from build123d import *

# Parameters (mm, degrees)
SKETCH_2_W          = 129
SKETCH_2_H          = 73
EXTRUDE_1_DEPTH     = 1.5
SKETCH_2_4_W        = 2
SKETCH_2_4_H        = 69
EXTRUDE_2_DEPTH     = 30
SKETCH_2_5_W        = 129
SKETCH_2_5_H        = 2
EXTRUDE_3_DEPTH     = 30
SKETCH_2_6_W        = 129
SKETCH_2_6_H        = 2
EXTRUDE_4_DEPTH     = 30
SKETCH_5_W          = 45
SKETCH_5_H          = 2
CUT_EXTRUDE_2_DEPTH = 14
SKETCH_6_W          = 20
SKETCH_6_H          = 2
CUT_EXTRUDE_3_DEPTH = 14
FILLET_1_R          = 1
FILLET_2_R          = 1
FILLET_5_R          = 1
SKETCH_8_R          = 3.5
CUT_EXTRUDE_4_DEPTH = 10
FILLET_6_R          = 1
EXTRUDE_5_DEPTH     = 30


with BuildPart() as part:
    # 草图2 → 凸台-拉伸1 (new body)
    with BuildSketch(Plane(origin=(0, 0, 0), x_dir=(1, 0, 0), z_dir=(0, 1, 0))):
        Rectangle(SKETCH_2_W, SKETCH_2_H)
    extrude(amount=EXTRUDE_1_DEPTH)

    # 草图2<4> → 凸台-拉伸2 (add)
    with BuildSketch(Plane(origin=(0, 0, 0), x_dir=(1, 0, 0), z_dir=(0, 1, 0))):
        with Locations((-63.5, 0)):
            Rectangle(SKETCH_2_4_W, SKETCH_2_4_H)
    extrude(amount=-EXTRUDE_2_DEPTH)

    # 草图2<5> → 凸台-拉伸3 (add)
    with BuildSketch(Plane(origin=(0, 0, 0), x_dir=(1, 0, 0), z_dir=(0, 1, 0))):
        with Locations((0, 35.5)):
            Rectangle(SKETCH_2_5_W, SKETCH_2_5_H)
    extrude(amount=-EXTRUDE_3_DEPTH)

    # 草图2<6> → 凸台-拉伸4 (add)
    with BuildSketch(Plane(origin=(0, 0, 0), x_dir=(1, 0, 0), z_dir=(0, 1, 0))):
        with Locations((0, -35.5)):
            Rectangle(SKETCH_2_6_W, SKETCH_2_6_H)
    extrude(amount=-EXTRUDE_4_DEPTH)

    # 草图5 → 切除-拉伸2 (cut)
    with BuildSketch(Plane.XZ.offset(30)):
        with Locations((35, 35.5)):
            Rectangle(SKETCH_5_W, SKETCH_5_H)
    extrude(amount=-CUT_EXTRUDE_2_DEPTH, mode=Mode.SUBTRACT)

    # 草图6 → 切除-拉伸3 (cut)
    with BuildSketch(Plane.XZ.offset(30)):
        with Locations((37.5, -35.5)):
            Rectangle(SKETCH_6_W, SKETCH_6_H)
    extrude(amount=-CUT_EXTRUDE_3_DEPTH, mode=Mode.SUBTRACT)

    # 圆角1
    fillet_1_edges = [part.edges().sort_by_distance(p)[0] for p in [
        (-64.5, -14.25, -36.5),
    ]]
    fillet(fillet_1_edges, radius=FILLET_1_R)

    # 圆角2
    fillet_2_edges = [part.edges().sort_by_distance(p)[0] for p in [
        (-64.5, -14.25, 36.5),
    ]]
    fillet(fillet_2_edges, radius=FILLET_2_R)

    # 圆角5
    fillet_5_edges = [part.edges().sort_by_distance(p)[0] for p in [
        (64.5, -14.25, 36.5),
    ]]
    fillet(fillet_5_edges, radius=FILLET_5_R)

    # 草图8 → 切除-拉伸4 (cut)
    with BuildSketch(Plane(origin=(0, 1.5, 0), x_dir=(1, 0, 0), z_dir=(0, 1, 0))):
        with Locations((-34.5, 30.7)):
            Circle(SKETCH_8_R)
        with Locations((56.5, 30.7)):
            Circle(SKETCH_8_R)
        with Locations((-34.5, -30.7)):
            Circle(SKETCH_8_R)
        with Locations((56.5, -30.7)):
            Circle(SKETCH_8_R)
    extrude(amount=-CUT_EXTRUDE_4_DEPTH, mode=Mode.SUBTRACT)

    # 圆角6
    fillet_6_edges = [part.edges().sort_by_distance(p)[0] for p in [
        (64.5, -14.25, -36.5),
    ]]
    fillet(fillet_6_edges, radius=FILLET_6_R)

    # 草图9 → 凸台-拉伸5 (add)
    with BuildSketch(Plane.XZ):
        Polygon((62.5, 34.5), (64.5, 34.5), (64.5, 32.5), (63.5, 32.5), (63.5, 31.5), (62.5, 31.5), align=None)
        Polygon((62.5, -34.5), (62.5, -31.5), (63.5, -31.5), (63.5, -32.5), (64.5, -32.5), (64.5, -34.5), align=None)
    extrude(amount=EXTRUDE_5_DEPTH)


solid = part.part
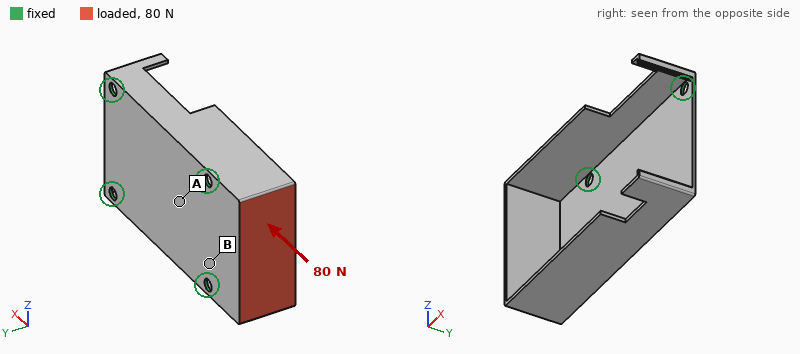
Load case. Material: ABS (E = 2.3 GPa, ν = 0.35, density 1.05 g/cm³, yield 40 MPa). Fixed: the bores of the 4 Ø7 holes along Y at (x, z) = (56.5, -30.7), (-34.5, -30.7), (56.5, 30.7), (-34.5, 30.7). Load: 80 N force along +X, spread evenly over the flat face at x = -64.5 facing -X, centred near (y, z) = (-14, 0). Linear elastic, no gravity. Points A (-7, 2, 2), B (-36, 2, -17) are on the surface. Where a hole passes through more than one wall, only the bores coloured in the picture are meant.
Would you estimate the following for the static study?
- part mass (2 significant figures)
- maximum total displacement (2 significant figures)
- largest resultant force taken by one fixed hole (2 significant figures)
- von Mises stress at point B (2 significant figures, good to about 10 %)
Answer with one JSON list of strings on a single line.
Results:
["34 g", "1.7 mm", "25 N", "1.3 MPa"]
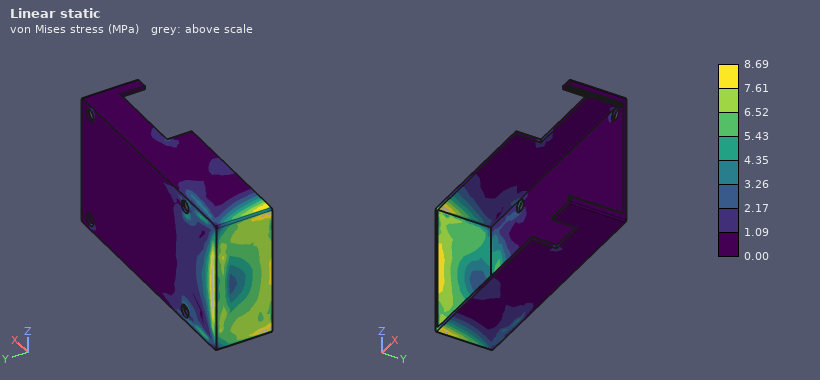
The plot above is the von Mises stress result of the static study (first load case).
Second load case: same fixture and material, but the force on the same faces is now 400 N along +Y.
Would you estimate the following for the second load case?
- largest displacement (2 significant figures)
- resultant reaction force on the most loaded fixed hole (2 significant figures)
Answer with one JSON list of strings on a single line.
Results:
["1.4 mm", "310 N"]
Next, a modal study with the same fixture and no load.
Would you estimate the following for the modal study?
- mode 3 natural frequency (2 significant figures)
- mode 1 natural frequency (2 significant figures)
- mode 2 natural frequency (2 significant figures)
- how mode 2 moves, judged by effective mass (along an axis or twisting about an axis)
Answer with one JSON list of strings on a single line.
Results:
["560 Hz", "330 Hz", "420 Hz", "along Z"]
